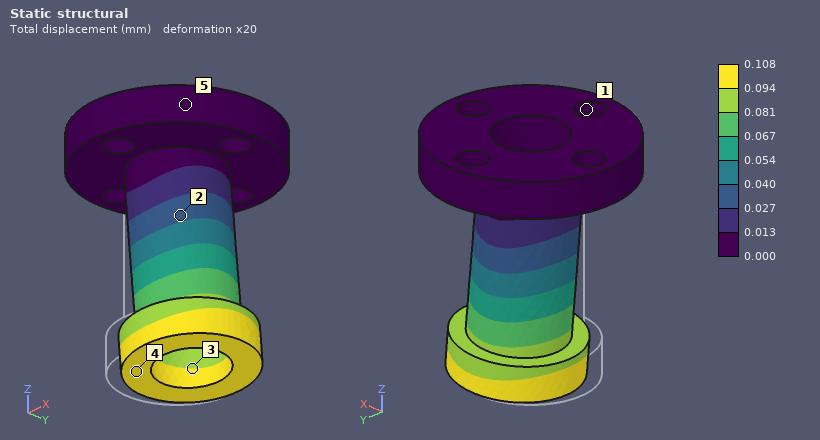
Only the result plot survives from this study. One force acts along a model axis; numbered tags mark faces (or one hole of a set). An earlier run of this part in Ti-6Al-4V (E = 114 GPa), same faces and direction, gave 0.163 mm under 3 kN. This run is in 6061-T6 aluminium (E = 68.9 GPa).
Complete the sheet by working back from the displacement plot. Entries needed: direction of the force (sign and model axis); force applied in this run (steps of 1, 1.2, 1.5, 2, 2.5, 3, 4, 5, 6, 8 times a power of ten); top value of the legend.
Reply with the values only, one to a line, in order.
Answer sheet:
+X
1.2 kN
0.108 mm
